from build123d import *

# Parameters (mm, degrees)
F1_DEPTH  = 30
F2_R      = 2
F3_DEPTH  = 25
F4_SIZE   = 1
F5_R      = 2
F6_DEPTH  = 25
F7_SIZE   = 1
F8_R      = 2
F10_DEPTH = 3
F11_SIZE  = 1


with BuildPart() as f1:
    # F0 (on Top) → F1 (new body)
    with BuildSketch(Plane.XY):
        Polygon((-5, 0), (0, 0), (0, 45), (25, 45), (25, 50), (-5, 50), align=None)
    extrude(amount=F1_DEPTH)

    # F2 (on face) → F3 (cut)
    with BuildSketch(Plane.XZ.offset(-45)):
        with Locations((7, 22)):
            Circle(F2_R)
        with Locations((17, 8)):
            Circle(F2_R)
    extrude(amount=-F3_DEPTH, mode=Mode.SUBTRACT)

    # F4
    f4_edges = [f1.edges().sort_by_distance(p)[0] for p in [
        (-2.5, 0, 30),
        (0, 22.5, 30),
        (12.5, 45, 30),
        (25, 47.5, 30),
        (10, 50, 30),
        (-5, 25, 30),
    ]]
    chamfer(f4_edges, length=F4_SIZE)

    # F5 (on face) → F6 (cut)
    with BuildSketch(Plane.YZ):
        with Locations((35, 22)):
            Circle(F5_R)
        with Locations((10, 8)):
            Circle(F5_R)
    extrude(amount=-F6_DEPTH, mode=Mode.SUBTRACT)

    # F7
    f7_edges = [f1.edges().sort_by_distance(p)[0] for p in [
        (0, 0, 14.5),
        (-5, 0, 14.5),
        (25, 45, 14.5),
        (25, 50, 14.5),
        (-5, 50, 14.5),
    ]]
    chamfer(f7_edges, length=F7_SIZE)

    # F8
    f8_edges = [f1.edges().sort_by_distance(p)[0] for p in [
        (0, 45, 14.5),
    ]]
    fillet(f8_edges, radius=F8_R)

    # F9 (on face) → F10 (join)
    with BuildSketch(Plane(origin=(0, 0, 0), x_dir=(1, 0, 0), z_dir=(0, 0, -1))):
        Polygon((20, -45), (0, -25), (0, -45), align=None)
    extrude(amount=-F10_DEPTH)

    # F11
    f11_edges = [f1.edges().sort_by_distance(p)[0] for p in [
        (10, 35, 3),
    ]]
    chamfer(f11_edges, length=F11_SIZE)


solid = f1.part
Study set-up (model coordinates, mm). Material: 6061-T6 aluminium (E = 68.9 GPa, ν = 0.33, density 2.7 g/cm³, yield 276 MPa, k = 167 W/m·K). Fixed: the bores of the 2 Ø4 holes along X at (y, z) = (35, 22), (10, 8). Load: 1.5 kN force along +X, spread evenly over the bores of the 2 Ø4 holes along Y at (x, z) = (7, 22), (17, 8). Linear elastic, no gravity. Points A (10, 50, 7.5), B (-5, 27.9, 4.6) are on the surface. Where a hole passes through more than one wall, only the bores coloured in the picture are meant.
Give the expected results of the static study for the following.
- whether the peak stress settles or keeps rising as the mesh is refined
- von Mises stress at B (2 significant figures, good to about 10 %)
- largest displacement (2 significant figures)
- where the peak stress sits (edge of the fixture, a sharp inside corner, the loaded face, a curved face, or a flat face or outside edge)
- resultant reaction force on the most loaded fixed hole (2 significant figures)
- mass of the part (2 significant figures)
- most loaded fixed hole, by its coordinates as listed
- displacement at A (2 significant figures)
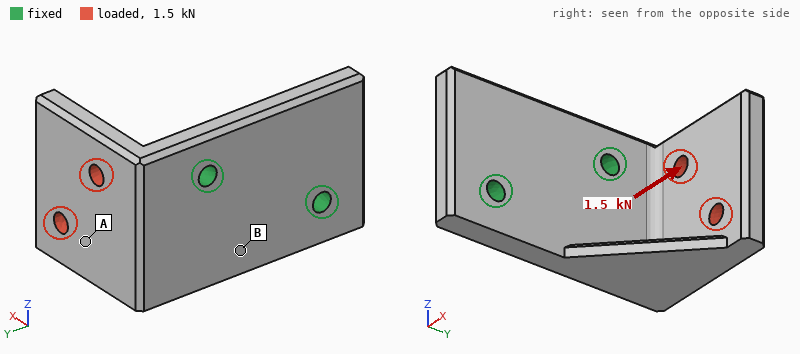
keeps rising
63 MPa
0.25 mm
edge of the fixture
1.7 kN
31 g
(35, 22)
0.16 mm
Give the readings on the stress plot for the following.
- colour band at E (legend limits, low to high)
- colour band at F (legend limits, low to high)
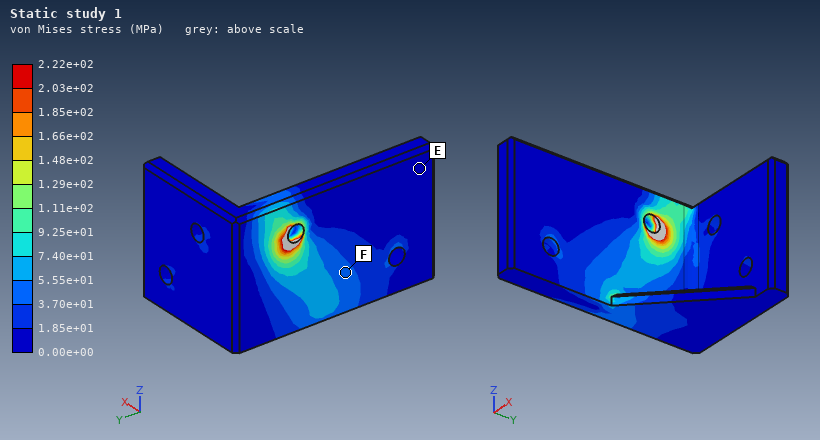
0.00e+00 to 1.85e+01 MPa
3.70e+01 to 5.55e+01 MPa
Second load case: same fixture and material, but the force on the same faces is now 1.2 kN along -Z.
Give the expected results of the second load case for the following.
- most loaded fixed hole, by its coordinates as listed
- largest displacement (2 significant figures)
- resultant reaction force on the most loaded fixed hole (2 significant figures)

(35, 22)
0.25 mm
1.5 kN
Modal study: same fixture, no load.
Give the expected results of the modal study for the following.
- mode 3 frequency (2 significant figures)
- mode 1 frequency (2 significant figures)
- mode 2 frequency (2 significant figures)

9900 Hz
3100 Hz
5000 Hz
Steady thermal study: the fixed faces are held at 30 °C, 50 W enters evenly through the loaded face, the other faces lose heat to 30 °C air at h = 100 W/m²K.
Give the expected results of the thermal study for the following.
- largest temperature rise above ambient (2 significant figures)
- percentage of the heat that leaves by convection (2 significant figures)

49 K
20 %
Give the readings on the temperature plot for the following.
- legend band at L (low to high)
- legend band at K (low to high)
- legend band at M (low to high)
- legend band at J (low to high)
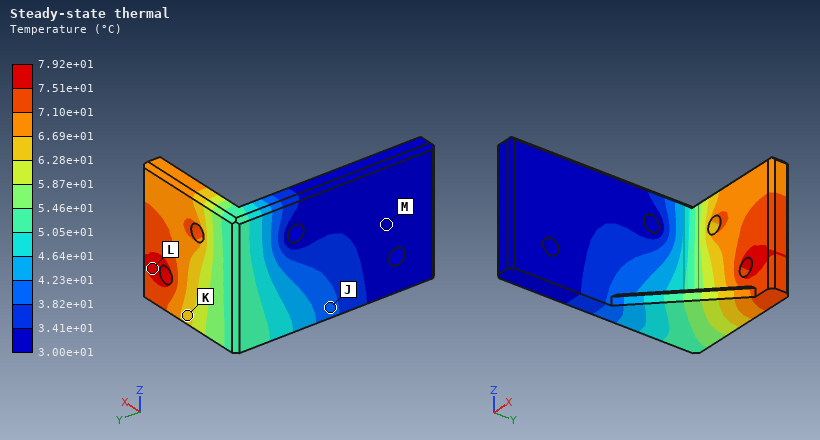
7.51e+01 to 7.92e+01 °C
6.28e+01 to 6.69e+01 °C
3.00e+01 to 3.41e+01 °C
3.82e+01 to 4.23e+01 °C
